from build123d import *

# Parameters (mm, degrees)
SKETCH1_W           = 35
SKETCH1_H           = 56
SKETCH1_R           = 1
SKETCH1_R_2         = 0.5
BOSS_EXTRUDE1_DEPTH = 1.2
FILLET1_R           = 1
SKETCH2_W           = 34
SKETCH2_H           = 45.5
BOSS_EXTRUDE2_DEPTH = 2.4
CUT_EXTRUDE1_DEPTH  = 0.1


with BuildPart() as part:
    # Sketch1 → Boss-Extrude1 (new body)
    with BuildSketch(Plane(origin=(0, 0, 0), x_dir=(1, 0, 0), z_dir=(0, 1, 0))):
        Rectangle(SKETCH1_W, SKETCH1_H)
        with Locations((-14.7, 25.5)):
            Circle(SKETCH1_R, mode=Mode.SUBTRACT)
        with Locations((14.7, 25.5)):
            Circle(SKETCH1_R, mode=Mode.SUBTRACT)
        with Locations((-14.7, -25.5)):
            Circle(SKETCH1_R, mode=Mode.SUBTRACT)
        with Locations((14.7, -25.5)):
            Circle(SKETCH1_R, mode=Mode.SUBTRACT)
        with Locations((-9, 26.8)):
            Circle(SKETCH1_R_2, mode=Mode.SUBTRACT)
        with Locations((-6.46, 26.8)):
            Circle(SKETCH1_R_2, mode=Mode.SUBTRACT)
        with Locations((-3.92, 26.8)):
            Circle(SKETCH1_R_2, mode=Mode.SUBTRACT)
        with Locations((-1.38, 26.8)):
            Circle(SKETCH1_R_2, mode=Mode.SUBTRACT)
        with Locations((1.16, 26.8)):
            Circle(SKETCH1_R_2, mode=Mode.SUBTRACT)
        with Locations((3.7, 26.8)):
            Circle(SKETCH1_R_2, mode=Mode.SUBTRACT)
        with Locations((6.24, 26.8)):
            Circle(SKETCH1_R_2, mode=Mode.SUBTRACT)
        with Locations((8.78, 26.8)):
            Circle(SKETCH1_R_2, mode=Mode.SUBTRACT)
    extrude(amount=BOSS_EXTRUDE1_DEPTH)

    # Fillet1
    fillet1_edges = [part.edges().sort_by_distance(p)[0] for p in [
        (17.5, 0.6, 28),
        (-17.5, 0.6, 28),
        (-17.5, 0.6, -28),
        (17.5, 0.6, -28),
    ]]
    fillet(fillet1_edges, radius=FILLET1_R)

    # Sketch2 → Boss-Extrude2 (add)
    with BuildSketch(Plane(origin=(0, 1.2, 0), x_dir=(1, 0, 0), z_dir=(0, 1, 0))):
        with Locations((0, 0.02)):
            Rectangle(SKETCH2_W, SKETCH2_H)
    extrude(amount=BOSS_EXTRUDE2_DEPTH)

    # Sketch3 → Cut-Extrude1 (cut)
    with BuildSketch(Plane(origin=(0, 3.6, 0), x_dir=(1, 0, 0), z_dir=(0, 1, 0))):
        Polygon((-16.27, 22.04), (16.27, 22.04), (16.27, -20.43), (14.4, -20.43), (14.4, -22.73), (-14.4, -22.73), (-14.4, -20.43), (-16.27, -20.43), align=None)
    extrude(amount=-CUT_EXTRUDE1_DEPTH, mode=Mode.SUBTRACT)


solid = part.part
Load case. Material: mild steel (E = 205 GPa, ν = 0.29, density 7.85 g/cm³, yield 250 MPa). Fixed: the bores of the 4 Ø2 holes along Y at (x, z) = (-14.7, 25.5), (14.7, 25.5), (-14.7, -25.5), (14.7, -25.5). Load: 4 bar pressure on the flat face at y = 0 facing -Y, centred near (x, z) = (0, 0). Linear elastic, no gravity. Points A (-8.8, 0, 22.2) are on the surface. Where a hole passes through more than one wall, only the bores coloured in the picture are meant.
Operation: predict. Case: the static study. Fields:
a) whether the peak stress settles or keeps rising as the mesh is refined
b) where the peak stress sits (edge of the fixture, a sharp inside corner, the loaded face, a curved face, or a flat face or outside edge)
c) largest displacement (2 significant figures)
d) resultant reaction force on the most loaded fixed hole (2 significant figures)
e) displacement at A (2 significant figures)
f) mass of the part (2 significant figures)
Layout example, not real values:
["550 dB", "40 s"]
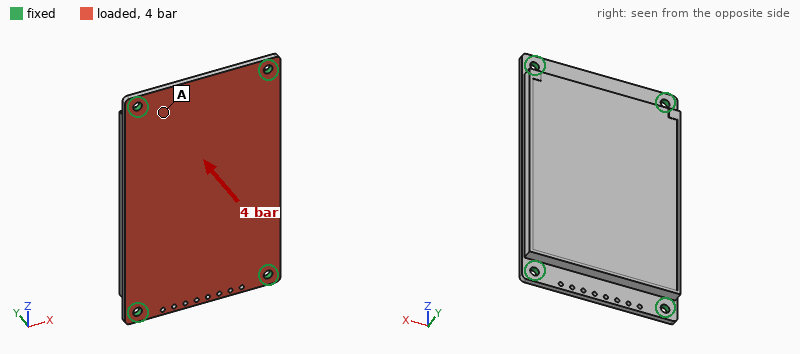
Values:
["keeps rising", "edge of the fixture", "28 µm", "440 N", "8.4 µm", "46 g"]
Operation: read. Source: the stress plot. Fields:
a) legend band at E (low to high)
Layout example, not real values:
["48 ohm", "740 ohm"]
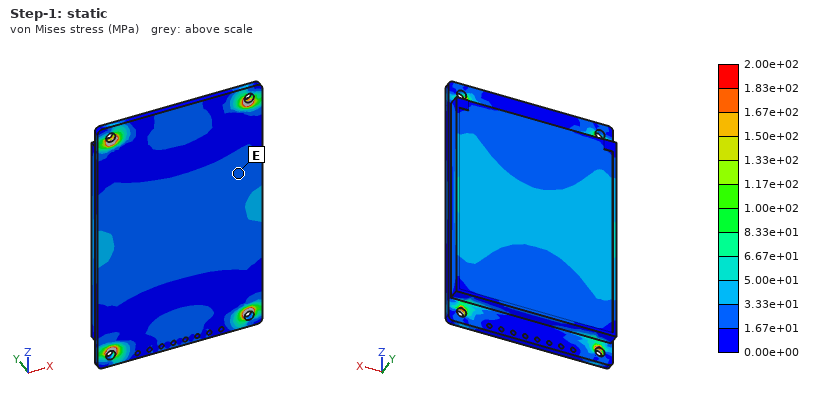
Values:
["1.67e+01 to 3.33e+01 MPa"]
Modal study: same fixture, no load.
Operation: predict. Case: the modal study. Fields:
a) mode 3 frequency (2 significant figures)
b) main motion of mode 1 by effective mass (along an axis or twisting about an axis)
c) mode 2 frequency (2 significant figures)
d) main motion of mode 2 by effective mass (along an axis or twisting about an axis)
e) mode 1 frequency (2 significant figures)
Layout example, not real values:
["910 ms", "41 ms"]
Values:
["10 kHz", "along Y", "7200 Hz", "twisting about Z", "4100 Hz"]
